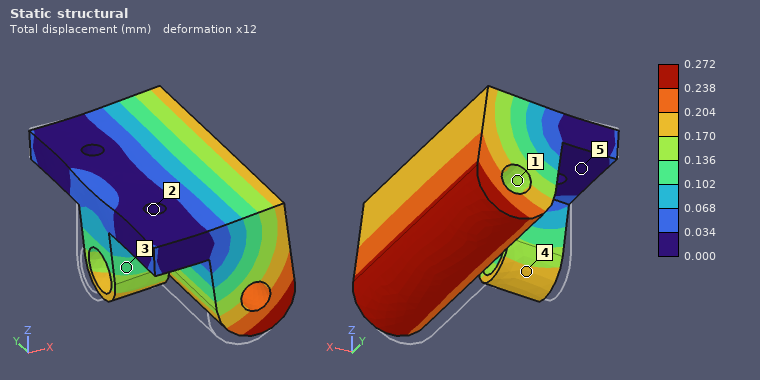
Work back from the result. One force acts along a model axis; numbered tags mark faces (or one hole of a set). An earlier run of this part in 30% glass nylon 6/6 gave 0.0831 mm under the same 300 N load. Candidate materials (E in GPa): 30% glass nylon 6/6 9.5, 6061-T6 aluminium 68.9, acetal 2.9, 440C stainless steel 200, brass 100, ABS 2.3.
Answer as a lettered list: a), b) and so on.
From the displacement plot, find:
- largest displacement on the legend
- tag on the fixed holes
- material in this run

a) 0.272 mm
b) 2
c) acetal
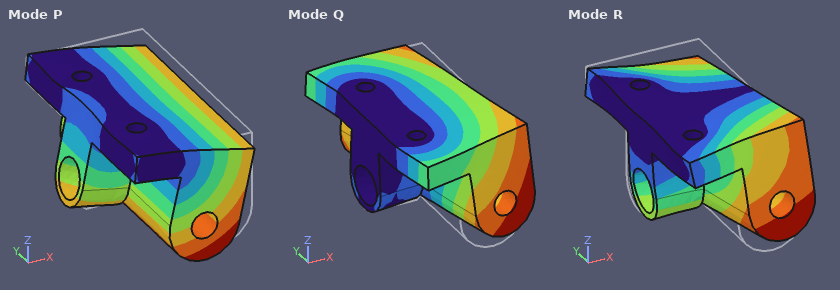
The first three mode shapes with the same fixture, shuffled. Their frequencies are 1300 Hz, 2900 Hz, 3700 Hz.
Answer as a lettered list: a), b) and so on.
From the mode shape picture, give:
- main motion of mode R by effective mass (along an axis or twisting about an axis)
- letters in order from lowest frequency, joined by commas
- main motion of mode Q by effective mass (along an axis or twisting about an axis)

a) along Y
b) P, R, Q
c) along Y
